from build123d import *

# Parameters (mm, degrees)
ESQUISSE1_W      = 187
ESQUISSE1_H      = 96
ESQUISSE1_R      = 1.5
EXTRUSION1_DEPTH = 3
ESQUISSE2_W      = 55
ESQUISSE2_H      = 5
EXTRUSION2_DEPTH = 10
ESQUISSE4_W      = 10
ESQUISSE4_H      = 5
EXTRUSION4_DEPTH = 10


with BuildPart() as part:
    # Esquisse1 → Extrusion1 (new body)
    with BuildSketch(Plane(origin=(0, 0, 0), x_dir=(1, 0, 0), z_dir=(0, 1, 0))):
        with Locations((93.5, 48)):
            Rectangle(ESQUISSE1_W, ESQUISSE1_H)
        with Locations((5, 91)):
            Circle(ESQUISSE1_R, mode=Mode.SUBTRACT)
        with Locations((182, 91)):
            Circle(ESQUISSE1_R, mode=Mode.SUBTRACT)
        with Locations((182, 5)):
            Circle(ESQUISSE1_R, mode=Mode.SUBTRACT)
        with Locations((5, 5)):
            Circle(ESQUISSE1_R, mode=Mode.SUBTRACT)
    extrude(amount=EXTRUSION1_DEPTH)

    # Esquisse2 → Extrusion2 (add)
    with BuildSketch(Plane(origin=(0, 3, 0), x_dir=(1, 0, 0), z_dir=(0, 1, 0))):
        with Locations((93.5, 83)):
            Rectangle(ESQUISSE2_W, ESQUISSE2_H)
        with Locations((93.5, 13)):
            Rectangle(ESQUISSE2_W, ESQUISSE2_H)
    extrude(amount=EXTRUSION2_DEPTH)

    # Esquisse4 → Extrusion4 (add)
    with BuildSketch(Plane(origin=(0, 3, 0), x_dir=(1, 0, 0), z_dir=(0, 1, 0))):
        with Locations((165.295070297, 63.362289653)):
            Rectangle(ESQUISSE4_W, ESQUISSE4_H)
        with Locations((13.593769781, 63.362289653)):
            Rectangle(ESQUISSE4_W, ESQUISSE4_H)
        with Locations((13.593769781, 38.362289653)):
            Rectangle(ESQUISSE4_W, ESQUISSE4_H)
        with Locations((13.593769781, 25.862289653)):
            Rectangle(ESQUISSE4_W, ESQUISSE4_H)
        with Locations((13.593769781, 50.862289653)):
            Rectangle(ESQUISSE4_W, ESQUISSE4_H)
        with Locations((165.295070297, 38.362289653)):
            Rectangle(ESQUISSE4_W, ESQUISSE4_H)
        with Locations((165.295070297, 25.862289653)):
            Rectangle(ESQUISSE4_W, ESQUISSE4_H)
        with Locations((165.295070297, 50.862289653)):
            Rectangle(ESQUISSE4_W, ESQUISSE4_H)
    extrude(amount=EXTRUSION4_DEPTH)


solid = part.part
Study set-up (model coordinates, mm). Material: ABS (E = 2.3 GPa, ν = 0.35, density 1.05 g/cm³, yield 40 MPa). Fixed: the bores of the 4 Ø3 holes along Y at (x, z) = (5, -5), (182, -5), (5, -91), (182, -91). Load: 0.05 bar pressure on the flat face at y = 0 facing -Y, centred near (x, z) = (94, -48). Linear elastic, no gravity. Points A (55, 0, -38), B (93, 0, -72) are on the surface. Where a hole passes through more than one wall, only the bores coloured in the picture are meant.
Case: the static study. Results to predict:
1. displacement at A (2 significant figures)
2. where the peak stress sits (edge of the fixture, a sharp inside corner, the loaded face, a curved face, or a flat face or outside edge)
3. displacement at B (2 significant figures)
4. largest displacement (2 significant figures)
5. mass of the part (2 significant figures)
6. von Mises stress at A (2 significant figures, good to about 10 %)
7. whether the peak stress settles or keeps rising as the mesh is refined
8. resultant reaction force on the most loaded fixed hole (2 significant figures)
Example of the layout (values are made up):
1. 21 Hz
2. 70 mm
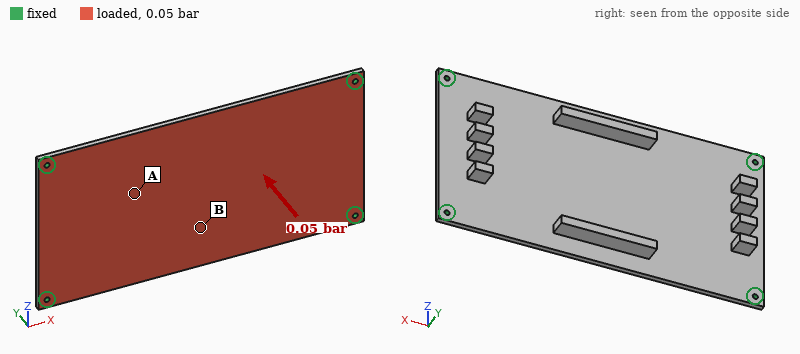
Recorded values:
1. 2.0 mm
2. edge of the fixture
3. 2.3 mm
4. 2.4 mm
5. 66 g
6. 3.3 MPa
7. keeps rising
8. 24 N
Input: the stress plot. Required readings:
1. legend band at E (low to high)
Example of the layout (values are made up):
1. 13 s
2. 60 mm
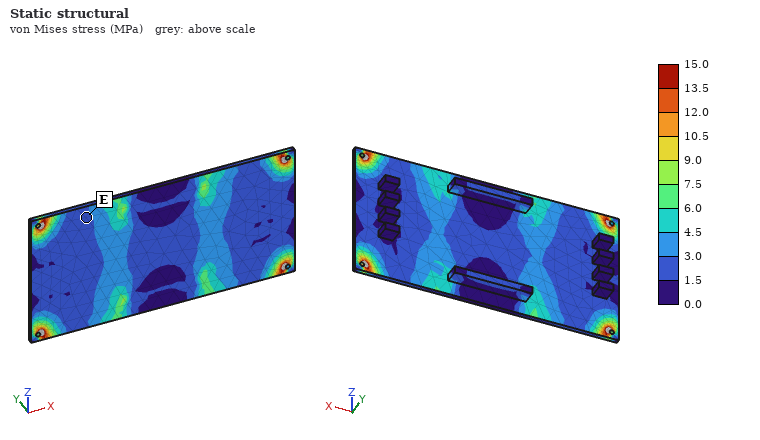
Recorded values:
1. 1.5 to 3.0 MPa
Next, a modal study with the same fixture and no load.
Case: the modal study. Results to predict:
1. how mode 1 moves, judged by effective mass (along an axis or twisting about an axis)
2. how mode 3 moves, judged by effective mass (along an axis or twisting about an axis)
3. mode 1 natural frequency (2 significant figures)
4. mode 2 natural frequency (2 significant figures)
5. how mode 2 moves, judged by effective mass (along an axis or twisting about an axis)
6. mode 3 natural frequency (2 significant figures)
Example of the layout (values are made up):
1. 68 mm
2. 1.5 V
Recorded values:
1. along Y
2. twisting about Z
3. 130 Hz
4. 220 Hz
5. twisting about X
6. 320 Hz
